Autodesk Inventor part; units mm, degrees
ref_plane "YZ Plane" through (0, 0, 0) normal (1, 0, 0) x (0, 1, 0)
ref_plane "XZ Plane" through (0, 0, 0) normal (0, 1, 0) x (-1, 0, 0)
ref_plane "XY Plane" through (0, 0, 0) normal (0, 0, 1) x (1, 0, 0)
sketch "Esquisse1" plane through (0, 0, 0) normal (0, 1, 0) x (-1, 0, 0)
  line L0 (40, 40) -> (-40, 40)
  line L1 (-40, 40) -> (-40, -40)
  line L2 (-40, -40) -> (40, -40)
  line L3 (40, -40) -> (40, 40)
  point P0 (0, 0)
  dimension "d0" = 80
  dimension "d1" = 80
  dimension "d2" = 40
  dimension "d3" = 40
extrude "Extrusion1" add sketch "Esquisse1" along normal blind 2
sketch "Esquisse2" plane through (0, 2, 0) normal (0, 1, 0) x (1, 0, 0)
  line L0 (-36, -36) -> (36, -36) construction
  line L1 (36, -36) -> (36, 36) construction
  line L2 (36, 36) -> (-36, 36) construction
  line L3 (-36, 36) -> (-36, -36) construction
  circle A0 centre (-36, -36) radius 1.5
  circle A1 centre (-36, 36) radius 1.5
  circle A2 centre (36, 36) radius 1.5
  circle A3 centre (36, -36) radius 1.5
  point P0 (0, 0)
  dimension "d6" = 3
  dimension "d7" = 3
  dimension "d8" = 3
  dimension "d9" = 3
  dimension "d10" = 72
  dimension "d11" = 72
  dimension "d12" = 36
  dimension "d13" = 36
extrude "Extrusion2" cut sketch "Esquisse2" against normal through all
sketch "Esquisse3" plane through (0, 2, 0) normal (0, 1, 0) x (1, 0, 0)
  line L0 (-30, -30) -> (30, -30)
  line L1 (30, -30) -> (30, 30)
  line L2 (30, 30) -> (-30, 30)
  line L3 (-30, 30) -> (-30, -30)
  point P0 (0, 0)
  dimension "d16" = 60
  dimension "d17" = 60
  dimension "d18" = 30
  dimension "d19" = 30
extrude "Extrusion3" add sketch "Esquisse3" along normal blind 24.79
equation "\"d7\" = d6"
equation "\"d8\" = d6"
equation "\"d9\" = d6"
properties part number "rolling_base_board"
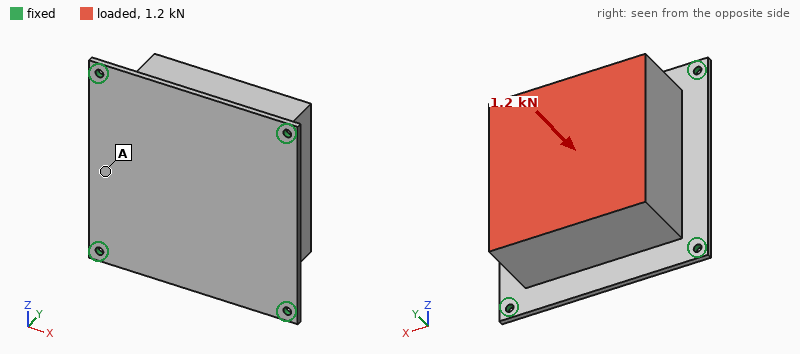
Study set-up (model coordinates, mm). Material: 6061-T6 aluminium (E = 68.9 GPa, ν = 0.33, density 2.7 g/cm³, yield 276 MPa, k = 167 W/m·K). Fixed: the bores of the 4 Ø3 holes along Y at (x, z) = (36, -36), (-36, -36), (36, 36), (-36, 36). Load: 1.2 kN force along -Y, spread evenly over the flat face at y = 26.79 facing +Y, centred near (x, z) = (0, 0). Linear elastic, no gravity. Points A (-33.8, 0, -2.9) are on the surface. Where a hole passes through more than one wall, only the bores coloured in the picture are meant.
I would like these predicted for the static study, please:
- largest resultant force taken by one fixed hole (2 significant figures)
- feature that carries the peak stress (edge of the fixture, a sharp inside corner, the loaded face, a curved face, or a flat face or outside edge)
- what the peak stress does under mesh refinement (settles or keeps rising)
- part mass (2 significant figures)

340 N
edge of the fixture
keeps rising
280 g
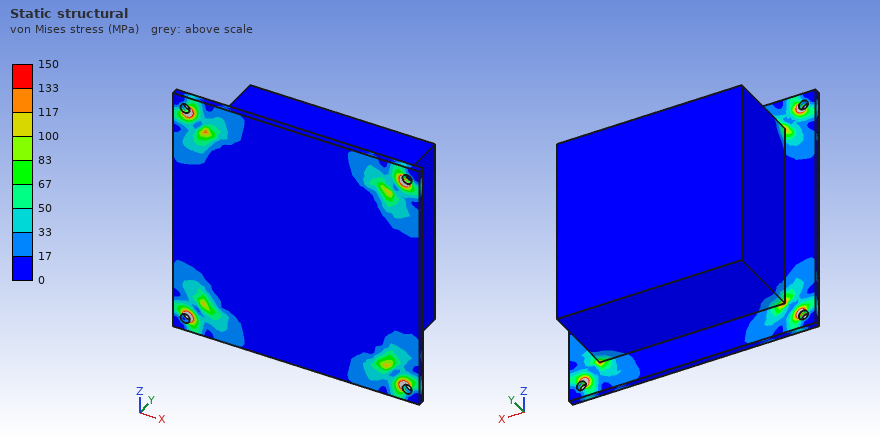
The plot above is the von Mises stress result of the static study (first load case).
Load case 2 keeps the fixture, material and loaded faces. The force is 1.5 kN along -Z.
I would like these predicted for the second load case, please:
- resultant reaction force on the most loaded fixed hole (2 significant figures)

520 N
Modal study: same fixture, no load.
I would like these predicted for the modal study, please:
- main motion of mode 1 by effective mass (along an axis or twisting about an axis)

along Y
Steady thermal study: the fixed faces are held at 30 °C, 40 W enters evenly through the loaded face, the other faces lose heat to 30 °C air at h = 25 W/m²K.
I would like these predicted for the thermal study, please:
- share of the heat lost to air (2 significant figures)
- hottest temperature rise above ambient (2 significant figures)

19 %
23 K
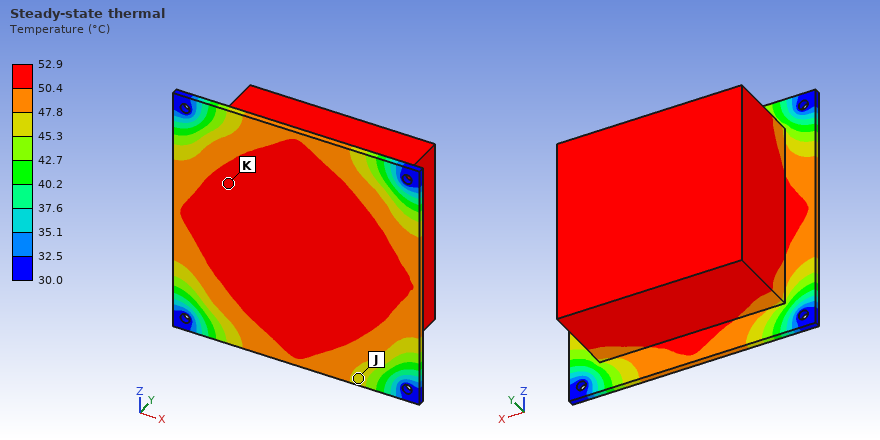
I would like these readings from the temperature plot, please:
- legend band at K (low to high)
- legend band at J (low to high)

50.4 to 52.9 °C
45.3 to 47.8 °C
